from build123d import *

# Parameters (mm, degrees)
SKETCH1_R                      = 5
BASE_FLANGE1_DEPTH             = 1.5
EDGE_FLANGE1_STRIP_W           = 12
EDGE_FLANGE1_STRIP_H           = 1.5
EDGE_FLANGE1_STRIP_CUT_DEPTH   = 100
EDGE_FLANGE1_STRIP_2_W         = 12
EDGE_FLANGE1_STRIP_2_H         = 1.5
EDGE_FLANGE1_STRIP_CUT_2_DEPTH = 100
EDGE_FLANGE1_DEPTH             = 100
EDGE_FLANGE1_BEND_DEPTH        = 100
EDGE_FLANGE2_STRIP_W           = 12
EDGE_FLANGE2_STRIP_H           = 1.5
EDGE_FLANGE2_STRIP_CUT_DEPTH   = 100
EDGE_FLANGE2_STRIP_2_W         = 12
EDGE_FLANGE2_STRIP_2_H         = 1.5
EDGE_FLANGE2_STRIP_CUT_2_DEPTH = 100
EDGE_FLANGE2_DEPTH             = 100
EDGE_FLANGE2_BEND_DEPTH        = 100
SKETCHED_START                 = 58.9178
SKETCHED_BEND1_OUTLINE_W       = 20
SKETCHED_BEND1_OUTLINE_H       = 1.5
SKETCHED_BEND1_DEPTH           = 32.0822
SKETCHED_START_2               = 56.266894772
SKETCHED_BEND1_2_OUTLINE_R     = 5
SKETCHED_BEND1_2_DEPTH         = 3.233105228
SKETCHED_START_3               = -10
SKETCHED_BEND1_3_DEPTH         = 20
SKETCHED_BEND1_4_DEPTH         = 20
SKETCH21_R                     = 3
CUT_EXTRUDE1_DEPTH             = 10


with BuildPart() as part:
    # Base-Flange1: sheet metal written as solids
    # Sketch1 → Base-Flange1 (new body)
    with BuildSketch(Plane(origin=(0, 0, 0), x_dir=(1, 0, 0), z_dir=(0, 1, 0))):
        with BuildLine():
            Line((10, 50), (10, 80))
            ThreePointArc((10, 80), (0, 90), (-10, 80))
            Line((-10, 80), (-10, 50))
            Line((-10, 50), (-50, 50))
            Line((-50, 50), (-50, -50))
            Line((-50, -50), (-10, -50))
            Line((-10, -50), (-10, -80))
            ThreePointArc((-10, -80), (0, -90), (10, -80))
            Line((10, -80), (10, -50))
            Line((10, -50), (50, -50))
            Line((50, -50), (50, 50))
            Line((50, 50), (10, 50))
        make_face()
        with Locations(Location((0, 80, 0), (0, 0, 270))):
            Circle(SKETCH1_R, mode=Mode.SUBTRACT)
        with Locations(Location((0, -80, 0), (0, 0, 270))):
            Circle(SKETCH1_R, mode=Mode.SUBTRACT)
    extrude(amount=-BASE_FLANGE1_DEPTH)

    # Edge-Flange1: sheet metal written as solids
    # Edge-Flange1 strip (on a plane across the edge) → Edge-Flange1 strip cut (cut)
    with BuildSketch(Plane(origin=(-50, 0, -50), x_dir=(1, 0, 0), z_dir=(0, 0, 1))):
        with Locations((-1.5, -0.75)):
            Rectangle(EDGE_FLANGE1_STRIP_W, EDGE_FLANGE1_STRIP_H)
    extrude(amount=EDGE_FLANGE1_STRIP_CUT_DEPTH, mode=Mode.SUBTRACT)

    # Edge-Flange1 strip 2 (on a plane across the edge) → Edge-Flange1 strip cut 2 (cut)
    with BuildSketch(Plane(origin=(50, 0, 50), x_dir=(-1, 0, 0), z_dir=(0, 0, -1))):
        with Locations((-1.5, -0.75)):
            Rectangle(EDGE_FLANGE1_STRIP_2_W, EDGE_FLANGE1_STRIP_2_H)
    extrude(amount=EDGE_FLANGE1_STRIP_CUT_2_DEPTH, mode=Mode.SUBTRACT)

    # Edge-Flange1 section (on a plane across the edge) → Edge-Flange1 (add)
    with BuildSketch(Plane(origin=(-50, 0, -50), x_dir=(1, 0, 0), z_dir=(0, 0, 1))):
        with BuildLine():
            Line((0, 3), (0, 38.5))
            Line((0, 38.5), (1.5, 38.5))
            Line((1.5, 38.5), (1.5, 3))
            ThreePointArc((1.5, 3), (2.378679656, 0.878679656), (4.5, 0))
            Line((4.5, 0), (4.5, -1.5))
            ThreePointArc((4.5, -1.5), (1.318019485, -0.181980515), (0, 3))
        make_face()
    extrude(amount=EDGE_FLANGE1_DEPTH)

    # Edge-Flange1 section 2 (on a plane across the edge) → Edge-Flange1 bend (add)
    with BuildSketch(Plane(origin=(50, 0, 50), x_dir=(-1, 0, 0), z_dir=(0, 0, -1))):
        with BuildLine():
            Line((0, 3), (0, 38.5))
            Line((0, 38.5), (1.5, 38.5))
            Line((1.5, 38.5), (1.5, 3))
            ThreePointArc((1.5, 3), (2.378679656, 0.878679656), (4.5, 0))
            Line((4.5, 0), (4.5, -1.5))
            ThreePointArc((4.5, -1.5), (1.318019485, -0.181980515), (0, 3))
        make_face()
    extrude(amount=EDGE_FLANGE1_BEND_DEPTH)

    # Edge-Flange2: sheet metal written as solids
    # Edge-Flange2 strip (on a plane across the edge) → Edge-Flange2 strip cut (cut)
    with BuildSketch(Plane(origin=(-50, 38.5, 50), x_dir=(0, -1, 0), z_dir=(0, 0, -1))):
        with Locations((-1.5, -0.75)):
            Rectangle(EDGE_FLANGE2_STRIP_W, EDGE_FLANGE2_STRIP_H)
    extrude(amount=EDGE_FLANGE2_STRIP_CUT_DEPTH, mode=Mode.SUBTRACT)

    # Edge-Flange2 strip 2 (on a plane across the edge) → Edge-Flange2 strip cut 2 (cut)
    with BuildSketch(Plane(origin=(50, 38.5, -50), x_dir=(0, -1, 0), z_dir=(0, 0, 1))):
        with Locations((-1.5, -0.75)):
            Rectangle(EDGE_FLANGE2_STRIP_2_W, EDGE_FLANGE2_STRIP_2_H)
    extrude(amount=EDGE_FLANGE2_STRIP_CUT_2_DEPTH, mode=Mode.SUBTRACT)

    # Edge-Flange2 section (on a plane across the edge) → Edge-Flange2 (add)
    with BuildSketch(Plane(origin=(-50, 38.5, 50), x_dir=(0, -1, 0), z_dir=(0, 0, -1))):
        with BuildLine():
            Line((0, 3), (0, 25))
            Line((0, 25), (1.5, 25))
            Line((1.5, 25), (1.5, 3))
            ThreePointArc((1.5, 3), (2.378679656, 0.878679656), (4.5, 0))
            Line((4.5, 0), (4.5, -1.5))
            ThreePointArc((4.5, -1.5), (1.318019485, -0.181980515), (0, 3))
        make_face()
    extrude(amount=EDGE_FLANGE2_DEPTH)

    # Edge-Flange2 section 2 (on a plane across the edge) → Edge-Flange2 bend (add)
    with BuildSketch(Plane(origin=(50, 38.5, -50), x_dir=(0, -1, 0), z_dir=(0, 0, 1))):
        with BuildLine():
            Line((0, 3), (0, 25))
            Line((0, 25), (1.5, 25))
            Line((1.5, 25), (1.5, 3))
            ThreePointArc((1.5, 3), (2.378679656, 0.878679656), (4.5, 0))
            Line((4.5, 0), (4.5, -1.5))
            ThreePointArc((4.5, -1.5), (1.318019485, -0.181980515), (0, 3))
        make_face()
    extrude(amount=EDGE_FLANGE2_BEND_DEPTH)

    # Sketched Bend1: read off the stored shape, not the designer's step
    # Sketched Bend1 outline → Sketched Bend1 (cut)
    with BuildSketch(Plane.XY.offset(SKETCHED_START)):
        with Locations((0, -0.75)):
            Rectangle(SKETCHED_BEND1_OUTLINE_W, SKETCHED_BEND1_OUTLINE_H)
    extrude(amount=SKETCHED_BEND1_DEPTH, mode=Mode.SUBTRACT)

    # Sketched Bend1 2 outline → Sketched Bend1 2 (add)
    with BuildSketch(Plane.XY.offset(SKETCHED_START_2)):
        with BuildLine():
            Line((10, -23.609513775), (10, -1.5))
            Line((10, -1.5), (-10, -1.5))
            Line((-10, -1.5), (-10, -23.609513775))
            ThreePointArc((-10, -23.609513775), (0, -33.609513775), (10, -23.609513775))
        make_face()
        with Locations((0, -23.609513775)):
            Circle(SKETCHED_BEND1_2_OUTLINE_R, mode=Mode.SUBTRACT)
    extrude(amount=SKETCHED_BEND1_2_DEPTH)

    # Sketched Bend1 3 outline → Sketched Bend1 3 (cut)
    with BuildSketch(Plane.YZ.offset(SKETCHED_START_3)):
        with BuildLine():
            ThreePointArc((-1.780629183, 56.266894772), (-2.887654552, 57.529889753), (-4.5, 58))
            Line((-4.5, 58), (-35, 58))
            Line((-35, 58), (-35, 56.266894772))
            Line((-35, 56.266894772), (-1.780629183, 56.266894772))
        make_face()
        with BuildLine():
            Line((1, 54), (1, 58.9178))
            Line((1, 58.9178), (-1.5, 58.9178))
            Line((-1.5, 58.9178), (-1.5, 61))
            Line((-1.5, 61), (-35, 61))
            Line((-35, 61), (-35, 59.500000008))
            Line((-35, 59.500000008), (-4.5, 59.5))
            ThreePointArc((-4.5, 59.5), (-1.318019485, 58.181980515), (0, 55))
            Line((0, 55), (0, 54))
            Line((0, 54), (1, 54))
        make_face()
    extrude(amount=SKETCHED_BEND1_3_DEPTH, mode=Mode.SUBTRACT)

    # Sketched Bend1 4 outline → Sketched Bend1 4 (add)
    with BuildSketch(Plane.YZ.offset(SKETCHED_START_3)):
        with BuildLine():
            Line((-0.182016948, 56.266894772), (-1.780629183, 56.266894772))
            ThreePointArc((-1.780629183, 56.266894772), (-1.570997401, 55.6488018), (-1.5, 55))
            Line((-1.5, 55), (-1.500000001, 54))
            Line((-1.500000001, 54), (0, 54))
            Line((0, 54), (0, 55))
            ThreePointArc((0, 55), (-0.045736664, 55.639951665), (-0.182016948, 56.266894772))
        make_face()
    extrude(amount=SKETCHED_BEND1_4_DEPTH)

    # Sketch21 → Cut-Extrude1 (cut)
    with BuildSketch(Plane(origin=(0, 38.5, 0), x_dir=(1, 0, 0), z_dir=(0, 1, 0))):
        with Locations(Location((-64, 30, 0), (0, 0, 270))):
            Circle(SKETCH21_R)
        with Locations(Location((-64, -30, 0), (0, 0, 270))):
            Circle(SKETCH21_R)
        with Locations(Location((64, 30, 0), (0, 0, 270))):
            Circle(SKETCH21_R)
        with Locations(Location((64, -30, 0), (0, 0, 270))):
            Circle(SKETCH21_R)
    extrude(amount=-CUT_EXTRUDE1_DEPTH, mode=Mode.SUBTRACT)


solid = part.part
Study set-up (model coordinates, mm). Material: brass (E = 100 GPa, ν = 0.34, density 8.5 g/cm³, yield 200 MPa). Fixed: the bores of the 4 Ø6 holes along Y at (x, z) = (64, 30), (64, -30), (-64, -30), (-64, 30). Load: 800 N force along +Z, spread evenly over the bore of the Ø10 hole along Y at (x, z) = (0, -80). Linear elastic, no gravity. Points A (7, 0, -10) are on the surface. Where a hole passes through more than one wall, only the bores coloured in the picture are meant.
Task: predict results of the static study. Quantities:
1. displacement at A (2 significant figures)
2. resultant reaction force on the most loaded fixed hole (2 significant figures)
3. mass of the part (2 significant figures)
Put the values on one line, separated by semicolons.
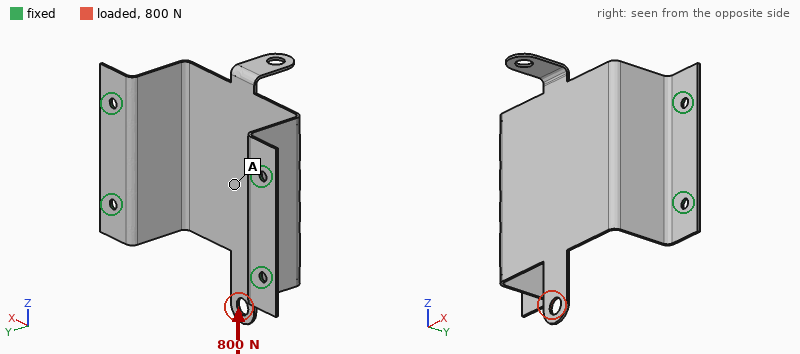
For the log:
0.15 mm; 340 N; 300 g
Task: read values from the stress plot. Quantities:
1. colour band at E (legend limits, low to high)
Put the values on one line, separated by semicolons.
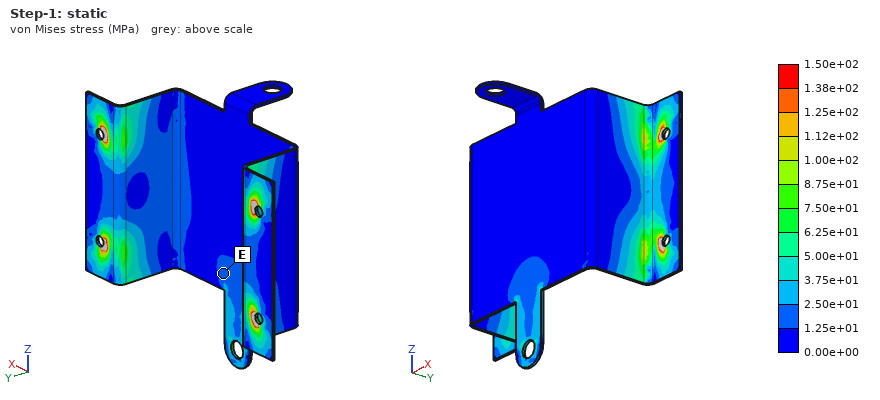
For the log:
1.25e+01 to 2.50e+01 MPa
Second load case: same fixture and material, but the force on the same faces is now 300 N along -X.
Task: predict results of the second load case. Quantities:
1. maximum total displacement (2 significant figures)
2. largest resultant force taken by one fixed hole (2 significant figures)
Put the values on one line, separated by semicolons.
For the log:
0.96 mm; 270 N
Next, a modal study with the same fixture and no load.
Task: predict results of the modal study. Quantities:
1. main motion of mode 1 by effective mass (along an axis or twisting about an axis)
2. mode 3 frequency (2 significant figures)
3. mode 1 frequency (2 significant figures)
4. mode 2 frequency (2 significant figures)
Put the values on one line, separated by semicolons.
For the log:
along X; 340 Hz; 250 Hz; 280 Hz
